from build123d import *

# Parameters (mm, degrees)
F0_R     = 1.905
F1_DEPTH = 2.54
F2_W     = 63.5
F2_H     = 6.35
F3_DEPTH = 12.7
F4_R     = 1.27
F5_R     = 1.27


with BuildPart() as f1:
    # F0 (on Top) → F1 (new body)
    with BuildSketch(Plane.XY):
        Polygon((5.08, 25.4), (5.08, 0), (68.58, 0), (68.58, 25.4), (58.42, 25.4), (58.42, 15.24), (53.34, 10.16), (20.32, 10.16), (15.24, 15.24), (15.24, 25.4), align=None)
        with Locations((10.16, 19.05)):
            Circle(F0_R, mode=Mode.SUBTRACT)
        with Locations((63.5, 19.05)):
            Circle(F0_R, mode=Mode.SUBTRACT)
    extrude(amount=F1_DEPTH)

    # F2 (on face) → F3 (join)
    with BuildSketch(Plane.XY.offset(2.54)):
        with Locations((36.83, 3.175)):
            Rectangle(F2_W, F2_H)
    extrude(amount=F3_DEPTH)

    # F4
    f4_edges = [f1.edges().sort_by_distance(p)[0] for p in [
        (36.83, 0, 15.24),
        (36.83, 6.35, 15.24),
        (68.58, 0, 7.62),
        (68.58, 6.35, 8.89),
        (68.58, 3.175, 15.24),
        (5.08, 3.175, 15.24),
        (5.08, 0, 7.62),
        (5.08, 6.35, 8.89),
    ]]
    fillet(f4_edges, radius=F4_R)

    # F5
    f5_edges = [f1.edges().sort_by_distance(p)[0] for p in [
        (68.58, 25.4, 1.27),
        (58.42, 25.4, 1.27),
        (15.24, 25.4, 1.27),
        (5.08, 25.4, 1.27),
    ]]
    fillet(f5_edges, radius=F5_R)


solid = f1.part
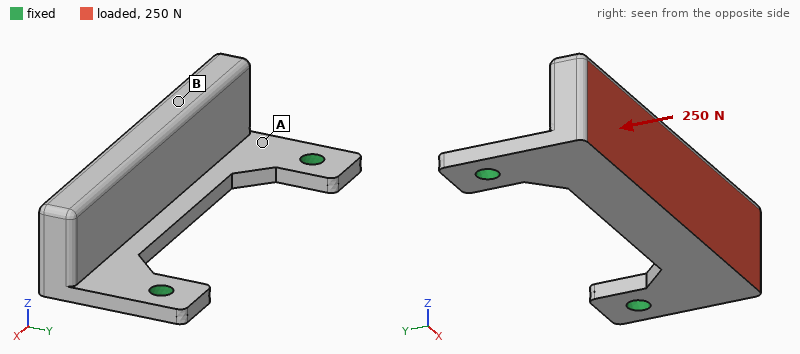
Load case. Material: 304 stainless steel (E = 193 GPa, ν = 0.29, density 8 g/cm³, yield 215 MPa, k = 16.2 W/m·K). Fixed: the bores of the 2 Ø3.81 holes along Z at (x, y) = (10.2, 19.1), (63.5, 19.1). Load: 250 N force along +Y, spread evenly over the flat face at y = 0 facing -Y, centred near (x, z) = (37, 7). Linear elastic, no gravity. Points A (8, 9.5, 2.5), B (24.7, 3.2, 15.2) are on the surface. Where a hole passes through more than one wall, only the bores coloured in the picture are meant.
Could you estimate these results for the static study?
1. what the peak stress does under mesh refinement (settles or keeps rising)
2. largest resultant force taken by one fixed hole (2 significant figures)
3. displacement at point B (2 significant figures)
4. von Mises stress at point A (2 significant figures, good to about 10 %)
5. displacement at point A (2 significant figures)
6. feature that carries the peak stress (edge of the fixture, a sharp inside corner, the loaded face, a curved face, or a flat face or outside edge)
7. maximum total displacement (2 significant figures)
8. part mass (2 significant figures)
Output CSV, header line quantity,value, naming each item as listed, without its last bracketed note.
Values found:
quantity,value
what the peak stress does under mesh refinement,keeps rising
largest resultant force taken by one fixed hole,140 N
displacement at point B,47 µm
von Mises stress at point A,47 MPa
displacement at point A,9.3 µm
feature that carries the peak stress,edge of the fixture
maximum total displacement,51 µm
part mass,60 g
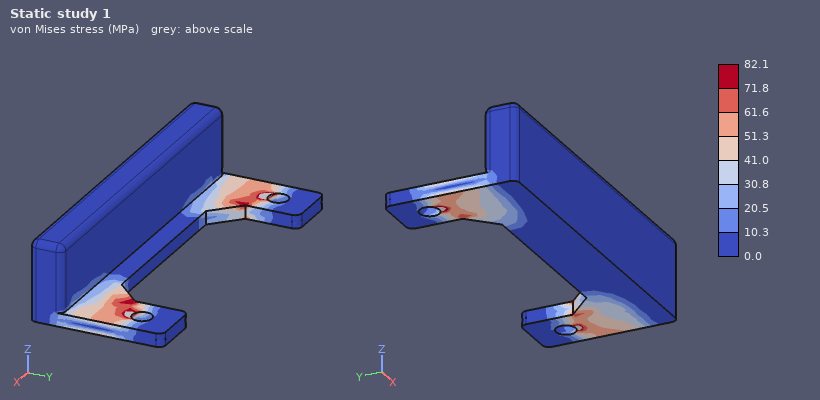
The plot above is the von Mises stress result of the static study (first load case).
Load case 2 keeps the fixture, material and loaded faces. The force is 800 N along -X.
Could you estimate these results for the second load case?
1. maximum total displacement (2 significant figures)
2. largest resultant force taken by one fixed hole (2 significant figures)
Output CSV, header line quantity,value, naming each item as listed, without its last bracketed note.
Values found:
quantity,value
maximum total displacement,11 µm
largest resultant force taken by one fixed hole,460 N
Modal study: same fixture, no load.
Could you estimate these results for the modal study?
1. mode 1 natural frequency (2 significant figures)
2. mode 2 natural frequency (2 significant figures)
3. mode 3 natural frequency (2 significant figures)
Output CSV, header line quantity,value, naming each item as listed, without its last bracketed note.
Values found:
quantity,value
mode 1 natural frequency,1300 Hz
mode 2 natural frequency,4400 Hz
mode 3 natural frequency,5700 Hz
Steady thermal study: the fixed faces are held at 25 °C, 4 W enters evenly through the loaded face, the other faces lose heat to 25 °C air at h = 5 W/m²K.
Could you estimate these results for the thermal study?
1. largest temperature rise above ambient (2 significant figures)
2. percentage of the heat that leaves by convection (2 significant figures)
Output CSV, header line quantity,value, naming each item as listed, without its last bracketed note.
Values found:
quantity,value
largest temperature rise above ambient,56 K
percentage of the heat that leaves by convection,16 %
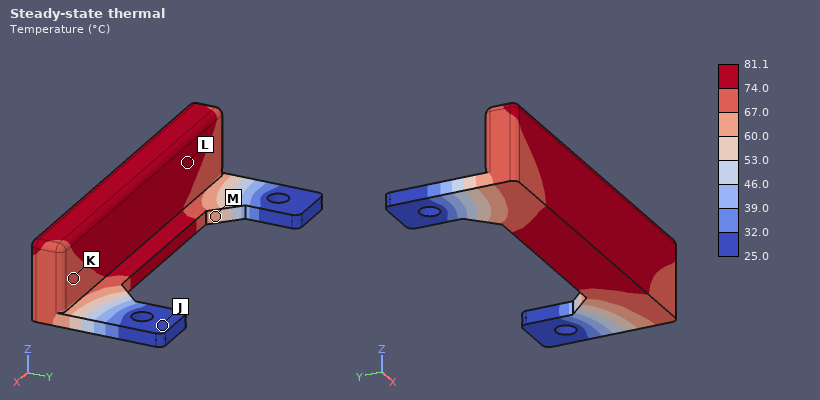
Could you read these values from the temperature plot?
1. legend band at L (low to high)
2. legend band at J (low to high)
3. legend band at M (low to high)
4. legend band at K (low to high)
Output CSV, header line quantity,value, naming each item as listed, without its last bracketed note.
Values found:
quantity,value
legend band at L,74.0 to 81.1 °C
legend band at J,25.0 to 32.0 °C
legend band at M,60.0 to 67.0 °C
legend band at K,67.0 to 74.0 °C
